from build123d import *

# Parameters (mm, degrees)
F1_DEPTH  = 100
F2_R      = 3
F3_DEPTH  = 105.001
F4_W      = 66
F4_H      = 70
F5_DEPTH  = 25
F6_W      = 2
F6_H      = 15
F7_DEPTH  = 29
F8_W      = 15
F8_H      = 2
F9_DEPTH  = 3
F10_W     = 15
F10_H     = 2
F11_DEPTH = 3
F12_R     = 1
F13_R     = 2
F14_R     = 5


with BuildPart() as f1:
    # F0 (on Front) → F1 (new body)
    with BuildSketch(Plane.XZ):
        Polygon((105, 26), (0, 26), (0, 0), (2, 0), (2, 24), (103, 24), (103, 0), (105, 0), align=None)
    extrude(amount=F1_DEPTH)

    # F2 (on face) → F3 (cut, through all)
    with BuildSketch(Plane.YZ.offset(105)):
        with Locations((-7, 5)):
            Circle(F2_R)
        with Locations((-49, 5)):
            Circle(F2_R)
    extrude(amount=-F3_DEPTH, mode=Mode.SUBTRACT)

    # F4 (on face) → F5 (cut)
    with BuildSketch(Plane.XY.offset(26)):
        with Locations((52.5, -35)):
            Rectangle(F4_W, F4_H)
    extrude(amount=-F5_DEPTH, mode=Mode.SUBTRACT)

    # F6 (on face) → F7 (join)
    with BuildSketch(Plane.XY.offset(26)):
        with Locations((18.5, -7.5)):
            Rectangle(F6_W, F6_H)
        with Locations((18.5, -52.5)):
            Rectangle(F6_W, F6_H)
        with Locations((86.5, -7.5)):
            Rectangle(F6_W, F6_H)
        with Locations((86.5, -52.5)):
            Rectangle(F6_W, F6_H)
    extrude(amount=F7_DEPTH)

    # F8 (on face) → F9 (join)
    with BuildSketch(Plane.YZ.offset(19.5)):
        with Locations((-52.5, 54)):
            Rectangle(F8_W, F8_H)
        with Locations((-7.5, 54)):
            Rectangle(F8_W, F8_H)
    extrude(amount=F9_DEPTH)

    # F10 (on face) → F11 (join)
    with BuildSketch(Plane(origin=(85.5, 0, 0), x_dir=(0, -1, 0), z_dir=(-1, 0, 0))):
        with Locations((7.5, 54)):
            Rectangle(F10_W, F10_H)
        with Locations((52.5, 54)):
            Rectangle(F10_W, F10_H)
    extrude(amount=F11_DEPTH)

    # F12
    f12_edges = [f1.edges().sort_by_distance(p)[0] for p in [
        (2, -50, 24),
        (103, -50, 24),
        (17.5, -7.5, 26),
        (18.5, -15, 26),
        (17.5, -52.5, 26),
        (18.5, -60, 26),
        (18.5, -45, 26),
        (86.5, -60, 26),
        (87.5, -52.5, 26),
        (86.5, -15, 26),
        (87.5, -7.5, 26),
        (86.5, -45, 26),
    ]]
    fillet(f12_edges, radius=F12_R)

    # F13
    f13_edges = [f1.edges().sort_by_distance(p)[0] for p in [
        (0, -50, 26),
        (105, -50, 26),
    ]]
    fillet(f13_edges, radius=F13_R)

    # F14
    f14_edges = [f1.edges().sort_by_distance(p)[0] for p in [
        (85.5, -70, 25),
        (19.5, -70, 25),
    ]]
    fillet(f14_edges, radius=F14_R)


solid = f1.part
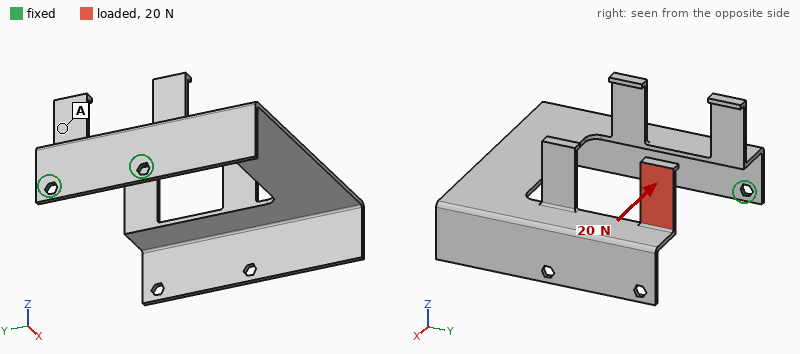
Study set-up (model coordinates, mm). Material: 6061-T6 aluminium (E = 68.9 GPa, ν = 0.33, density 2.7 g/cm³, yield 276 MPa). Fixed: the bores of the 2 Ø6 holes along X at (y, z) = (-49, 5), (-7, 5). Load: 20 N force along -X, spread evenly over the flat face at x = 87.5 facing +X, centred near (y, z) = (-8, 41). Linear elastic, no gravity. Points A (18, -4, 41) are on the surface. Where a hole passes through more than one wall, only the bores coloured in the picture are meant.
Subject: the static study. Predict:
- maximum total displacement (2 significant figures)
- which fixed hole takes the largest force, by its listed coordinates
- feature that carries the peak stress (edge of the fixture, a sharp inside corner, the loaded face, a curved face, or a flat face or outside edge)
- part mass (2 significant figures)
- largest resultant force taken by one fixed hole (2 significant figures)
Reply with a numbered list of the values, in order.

1. 1.7 mm
2. (-7, 5)
3. a curved face
4. 67 g
5. 17 N
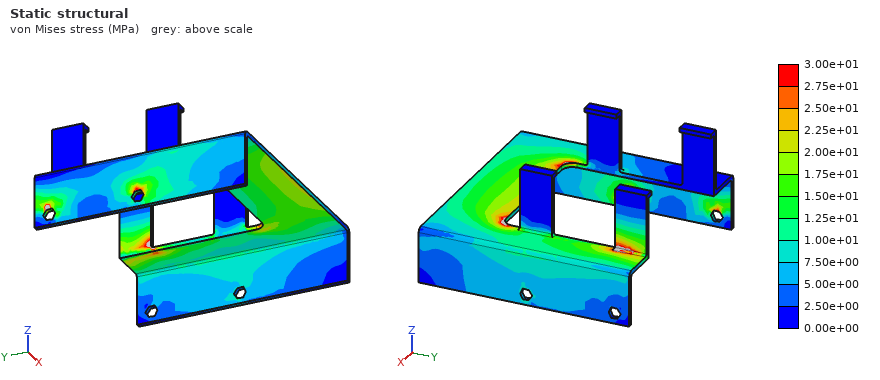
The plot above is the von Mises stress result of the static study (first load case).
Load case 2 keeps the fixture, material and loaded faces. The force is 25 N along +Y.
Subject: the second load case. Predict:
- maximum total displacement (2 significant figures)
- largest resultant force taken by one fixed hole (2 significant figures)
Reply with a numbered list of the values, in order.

1. 1.8 mm
2. 54 N
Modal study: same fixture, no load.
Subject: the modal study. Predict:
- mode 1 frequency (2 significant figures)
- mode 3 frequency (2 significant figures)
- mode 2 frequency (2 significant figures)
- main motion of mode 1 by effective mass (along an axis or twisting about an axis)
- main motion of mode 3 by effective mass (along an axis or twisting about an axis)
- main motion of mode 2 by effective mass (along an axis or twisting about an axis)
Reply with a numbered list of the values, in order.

1. 51 Hz
2. 240 Hz
3. 140 Hz
4. along Z
5. along Y
6. twisting about X
